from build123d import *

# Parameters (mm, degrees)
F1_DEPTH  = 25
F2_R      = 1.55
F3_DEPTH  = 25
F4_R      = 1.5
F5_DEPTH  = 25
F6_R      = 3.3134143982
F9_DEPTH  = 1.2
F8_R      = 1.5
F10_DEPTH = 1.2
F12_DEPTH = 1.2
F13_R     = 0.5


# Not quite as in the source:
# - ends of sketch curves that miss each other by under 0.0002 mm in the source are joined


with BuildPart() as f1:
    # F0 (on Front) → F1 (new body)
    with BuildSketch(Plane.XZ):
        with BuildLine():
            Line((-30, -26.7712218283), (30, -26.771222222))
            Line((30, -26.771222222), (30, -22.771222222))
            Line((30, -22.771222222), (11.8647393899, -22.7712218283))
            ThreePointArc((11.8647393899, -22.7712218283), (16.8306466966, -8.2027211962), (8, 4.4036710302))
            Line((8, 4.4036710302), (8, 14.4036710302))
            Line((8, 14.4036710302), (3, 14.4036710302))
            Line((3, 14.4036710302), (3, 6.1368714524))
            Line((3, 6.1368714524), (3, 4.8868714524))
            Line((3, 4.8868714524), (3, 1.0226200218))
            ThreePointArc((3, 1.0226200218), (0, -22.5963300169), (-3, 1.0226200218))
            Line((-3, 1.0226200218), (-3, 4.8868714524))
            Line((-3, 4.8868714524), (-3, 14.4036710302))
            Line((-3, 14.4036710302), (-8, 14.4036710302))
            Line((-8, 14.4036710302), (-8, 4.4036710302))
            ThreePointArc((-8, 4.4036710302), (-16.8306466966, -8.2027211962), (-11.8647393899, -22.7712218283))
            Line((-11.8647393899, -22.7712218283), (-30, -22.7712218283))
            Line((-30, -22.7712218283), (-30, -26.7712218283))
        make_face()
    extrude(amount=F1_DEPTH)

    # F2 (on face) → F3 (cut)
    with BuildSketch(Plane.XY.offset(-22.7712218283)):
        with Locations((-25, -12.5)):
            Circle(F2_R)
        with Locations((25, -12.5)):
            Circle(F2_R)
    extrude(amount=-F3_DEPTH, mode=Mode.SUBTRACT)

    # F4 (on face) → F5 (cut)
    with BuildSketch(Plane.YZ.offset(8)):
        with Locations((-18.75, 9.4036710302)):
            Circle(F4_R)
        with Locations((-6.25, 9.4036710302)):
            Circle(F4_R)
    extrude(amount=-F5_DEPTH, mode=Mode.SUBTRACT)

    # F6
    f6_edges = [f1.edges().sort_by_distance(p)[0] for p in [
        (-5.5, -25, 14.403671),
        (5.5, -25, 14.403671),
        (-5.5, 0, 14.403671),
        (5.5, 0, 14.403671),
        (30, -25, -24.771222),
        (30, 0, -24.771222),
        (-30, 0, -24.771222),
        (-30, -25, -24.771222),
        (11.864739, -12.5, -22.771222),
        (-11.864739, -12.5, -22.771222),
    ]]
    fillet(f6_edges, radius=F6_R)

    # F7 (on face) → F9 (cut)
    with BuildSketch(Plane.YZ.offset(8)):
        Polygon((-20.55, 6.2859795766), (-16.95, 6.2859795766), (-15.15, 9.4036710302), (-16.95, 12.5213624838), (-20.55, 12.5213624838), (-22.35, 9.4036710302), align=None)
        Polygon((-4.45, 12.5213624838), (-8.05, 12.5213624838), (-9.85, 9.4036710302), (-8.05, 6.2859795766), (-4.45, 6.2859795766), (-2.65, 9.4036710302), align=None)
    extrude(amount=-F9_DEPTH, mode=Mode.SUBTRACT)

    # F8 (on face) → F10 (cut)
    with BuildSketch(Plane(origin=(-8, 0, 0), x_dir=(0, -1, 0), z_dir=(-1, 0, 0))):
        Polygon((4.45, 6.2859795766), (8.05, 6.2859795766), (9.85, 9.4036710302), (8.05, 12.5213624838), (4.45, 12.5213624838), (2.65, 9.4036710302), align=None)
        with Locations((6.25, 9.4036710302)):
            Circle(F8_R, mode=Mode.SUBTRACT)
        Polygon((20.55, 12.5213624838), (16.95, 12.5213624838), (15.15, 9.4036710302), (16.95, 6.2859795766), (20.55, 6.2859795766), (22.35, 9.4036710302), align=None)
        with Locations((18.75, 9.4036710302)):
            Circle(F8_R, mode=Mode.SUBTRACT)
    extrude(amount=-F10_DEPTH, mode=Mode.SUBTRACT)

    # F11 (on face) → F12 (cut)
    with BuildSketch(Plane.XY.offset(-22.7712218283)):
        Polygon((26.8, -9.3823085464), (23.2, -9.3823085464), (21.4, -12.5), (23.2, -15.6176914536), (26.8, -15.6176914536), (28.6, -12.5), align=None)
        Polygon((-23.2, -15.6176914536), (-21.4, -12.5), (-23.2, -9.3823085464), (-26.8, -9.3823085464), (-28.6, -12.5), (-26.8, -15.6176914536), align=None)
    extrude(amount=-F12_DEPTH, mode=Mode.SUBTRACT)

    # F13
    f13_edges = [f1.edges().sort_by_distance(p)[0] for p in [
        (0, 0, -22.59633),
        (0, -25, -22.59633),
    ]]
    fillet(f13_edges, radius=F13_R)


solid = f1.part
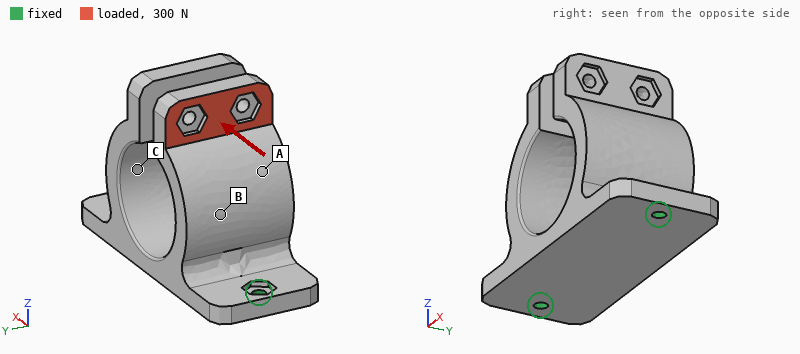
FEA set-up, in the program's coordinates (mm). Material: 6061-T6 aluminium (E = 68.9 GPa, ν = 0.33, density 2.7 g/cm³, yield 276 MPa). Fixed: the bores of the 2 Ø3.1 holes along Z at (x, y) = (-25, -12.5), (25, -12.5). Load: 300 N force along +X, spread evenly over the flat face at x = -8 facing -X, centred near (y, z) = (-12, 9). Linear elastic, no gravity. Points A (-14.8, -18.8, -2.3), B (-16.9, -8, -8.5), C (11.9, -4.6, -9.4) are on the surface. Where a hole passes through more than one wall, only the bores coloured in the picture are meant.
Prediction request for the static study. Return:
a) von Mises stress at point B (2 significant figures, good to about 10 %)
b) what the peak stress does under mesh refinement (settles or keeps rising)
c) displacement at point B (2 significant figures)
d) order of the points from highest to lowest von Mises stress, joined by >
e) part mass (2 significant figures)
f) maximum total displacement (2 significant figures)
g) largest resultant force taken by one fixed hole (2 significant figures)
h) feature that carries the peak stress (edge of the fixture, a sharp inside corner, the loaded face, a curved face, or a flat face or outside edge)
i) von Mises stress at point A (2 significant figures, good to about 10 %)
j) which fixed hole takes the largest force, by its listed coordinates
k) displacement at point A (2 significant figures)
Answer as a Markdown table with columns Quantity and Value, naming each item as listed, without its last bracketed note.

| Quantity | Value |
|---|---|
| von Mises stress at point B | 42 MPa |
| what the peak stress does under mesh refinement | keeps rising |
| displacement at point B | 0.069 mm |
| order of the points from highest to lowest von Mises stress, joined by > | B > A > C |
| part mass | 45 g |
| maximum total displacement | 0.30 mm |
| largest resultant force taken by one fixed hole | 450 N |
| feature that carries the peak stress | edge of the fixture |
| von Mises stress at point A | 31 MPa |
| which fixed hole takes the largest force, by its listed coordinates | (25, -12.5) |
| displacement at point A | 0.12 mm |
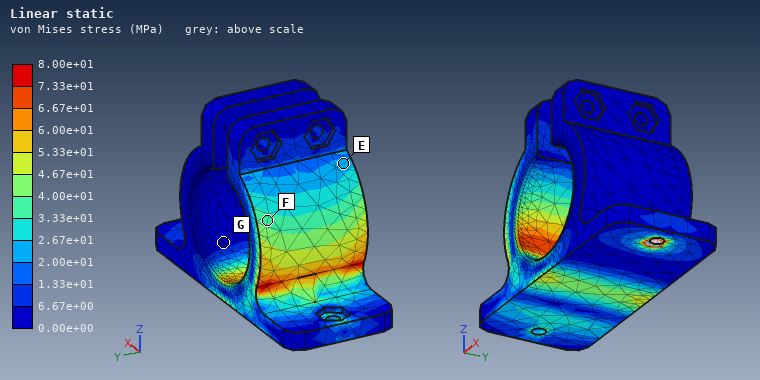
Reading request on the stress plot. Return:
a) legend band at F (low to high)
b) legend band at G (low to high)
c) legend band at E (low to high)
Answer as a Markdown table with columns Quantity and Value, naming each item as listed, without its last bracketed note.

| Quantity | Value |
|---|---|
| legend band at F | 3.33e+01 to 4.00e+01 MPa |
| legend band at G | 0.00e+00 to 6.67e+00 MPa |
| legend band at E | 2.00e+01 to 2.67e+01 MPa |
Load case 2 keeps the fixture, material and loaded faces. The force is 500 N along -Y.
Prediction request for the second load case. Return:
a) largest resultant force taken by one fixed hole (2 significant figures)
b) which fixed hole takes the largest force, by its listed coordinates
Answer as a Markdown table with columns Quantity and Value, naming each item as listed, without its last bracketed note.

| Quantity | Value |
|---|---|
| largest resultant force taken by one fixed hole | 330 N |
| which fixed hole takes the largest force, by its listed coordinates | (-25, -12.5) |
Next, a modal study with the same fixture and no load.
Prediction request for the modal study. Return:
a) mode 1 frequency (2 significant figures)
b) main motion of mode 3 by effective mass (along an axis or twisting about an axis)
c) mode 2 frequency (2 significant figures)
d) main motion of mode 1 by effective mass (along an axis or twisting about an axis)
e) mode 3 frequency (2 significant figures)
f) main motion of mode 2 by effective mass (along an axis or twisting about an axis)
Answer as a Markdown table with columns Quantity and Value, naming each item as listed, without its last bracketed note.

| Quantity | Value |
|---|---|
| mode 1 frequency | 1600 Hz |
| main motion of mode 3 by effective mass | along X |
| mode 2 frequency | 2000 Hz |
| main motion of mode 1 by effective mass | along Y |
| mode 3 frequency | 2900 Hz |
| main motion of mode 2 by effective mass | along Z |
